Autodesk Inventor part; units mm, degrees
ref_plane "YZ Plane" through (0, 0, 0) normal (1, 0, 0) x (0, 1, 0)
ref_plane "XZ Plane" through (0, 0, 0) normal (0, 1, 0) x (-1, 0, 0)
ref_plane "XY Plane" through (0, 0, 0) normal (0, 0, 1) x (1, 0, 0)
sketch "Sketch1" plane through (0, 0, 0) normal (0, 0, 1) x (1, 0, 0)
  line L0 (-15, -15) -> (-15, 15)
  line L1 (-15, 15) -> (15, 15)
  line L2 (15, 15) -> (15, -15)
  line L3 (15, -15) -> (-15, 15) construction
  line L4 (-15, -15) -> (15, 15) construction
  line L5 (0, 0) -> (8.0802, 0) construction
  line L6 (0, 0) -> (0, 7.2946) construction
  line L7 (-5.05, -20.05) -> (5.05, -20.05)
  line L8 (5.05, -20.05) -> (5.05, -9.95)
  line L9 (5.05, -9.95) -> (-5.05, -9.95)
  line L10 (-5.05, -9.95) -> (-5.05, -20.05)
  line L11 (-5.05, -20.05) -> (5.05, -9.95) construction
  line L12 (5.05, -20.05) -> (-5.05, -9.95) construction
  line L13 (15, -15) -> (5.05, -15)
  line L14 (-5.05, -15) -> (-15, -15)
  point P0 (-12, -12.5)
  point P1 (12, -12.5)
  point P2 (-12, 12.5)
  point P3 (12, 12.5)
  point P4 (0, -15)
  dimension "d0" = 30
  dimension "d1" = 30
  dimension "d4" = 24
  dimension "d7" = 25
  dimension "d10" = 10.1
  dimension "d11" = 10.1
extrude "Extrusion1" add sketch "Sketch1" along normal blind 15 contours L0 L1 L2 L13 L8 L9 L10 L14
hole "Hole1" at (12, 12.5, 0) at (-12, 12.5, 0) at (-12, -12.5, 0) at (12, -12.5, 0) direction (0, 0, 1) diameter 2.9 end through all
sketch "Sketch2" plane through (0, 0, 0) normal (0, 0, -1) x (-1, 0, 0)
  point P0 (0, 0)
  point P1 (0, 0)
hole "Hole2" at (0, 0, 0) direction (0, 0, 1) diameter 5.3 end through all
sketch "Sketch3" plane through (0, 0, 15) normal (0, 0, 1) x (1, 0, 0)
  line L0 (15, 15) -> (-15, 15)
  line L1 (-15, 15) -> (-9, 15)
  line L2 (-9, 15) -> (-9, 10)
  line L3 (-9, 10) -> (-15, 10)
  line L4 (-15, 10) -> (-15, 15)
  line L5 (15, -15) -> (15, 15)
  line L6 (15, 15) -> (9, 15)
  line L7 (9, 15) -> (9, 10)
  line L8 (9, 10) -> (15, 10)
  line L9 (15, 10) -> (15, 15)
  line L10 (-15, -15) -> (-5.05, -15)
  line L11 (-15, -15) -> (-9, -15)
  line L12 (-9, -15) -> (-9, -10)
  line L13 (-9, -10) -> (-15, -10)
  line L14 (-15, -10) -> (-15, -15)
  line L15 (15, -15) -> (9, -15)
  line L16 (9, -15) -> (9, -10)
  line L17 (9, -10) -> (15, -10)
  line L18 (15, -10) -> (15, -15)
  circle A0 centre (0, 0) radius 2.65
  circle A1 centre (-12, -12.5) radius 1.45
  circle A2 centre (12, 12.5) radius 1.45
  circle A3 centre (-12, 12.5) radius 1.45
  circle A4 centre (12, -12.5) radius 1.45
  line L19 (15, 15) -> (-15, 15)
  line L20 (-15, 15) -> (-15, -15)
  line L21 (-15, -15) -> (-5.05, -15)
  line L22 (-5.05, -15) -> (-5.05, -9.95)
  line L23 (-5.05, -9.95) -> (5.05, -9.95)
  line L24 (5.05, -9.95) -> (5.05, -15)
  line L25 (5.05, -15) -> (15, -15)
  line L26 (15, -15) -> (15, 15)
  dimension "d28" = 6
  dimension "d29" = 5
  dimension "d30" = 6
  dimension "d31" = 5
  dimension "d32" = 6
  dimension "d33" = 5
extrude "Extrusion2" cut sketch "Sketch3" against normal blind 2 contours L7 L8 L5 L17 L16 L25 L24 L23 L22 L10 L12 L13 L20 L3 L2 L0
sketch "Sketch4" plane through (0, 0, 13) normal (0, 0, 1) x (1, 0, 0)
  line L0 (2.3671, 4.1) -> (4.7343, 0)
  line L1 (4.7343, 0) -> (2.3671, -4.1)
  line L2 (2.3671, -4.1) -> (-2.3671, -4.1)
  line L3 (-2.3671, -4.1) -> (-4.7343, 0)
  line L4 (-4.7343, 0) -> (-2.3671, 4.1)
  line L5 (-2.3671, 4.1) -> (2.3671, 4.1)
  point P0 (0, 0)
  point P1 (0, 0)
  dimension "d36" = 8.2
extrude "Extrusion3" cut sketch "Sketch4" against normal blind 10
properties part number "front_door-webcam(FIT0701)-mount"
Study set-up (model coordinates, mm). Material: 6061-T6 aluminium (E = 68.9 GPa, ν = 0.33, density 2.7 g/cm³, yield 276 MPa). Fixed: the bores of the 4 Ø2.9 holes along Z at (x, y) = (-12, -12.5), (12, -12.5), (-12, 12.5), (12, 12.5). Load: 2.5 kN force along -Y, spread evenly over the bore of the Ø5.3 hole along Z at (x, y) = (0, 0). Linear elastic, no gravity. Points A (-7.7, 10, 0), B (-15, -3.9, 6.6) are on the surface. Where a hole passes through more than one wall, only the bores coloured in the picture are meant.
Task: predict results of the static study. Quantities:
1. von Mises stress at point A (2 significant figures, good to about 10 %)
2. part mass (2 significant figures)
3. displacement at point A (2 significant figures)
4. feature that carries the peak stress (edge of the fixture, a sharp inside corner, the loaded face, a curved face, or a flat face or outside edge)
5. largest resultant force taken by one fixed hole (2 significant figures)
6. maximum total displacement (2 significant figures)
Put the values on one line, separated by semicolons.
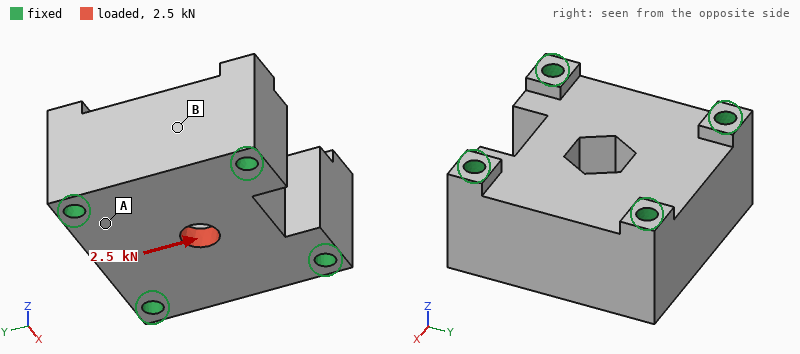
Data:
15 MPa; 28 g; 1.1 µm; a sharp inside corner; 770 N; 6.4 µm
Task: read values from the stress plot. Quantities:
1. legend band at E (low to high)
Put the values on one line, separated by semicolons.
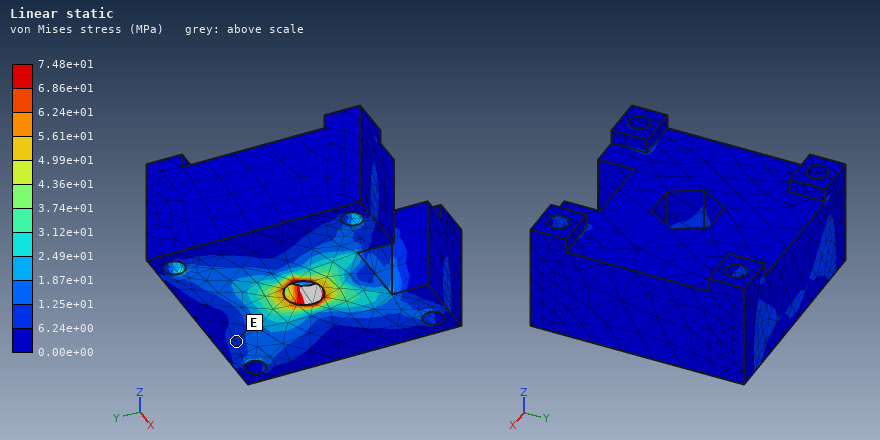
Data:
6.24e+00 to 1.25e+01 MPa
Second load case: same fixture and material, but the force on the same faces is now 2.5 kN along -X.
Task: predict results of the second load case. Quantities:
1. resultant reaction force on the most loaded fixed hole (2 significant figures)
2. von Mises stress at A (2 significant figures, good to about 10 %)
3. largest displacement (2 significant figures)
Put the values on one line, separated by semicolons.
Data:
820 N; 13 MPa; 6.1 µm
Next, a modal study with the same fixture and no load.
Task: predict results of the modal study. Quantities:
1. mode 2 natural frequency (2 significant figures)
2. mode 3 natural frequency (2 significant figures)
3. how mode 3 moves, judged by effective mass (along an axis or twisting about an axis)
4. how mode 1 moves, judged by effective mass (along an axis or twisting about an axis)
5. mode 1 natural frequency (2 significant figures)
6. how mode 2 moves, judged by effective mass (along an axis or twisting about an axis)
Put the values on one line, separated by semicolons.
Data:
50 kHz; 54 kHz; twisting about Y; along Z; 42 kHz; along X
